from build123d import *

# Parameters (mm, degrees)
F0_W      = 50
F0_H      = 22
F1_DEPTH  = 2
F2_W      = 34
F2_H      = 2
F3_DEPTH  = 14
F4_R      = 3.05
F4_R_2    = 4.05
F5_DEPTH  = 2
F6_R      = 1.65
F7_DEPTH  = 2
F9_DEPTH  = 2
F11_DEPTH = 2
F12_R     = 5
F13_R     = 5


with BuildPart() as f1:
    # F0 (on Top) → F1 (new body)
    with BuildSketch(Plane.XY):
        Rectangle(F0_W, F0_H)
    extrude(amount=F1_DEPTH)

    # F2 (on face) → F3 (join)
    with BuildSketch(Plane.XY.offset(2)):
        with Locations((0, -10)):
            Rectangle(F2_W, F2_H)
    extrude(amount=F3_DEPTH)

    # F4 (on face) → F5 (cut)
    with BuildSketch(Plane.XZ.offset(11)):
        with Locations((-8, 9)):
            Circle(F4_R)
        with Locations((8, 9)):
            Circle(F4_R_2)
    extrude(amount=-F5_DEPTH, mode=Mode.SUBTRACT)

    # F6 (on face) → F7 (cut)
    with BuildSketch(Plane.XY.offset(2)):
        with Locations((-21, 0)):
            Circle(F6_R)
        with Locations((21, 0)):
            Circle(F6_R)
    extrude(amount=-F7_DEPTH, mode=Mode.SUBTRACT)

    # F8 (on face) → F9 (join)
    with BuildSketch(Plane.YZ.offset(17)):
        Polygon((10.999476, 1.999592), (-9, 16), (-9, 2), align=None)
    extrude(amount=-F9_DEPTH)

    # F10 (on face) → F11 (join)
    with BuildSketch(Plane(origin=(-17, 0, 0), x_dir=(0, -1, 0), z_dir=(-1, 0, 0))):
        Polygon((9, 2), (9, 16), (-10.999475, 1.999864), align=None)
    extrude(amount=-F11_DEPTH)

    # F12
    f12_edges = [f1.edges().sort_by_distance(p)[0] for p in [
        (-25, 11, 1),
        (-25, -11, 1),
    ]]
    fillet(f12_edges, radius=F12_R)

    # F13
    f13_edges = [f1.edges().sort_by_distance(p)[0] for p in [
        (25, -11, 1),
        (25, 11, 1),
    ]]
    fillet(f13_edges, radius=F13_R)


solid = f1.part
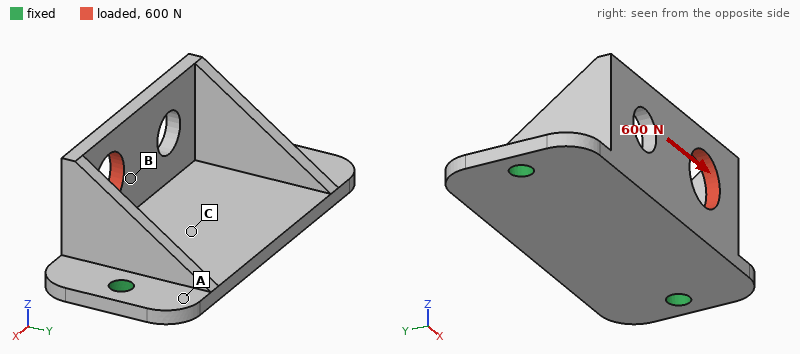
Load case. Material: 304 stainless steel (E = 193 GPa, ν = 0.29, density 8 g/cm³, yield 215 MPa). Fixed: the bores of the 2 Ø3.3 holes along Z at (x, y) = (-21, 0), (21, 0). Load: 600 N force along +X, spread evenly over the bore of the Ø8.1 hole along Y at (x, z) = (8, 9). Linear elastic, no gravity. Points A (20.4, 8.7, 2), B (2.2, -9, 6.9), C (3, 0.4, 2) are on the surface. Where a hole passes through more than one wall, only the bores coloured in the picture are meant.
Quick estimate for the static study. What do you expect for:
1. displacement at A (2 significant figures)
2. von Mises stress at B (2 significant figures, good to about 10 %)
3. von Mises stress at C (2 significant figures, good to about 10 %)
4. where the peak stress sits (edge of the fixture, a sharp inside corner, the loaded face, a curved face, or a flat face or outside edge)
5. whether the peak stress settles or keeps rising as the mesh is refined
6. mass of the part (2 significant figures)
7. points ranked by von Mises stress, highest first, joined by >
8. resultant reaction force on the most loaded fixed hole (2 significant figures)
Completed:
3.6 µm
30 MPa
17 MPa
edge of the fixture
keeps rising
28 g
B > C > A
360 N
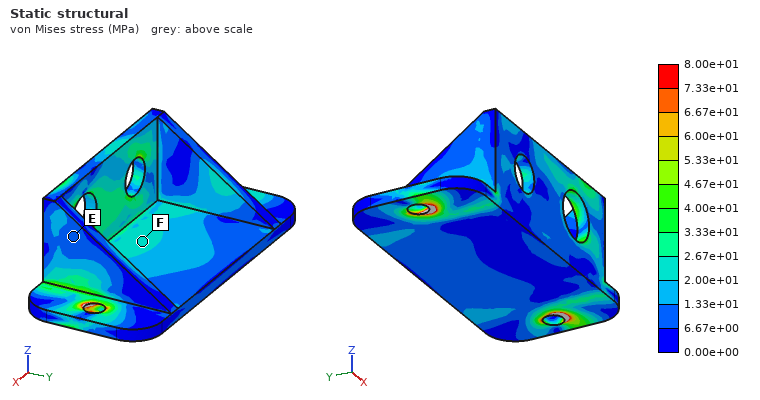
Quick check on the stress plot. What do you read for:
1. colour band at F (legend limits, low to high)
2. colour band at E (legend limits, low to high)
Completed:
2.00e+01 to 2.67e+01 MPa
6.67e+00 to 1.33e+01 MPa
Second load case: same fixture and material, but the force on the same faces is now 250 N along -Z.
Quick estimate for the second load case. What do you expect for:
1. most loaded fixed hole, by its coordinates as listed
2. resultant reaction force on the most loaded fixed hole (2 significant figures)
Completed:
(21, 0)
190 N
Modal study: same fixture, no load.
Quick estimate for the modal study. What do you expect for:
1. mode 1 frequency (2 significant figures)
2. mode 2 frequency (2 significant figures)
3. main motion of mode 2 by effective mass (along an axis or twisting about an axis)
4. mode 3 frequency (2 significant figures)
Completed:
4600 Hz
7300 Hz
along Z
8300 Hz
